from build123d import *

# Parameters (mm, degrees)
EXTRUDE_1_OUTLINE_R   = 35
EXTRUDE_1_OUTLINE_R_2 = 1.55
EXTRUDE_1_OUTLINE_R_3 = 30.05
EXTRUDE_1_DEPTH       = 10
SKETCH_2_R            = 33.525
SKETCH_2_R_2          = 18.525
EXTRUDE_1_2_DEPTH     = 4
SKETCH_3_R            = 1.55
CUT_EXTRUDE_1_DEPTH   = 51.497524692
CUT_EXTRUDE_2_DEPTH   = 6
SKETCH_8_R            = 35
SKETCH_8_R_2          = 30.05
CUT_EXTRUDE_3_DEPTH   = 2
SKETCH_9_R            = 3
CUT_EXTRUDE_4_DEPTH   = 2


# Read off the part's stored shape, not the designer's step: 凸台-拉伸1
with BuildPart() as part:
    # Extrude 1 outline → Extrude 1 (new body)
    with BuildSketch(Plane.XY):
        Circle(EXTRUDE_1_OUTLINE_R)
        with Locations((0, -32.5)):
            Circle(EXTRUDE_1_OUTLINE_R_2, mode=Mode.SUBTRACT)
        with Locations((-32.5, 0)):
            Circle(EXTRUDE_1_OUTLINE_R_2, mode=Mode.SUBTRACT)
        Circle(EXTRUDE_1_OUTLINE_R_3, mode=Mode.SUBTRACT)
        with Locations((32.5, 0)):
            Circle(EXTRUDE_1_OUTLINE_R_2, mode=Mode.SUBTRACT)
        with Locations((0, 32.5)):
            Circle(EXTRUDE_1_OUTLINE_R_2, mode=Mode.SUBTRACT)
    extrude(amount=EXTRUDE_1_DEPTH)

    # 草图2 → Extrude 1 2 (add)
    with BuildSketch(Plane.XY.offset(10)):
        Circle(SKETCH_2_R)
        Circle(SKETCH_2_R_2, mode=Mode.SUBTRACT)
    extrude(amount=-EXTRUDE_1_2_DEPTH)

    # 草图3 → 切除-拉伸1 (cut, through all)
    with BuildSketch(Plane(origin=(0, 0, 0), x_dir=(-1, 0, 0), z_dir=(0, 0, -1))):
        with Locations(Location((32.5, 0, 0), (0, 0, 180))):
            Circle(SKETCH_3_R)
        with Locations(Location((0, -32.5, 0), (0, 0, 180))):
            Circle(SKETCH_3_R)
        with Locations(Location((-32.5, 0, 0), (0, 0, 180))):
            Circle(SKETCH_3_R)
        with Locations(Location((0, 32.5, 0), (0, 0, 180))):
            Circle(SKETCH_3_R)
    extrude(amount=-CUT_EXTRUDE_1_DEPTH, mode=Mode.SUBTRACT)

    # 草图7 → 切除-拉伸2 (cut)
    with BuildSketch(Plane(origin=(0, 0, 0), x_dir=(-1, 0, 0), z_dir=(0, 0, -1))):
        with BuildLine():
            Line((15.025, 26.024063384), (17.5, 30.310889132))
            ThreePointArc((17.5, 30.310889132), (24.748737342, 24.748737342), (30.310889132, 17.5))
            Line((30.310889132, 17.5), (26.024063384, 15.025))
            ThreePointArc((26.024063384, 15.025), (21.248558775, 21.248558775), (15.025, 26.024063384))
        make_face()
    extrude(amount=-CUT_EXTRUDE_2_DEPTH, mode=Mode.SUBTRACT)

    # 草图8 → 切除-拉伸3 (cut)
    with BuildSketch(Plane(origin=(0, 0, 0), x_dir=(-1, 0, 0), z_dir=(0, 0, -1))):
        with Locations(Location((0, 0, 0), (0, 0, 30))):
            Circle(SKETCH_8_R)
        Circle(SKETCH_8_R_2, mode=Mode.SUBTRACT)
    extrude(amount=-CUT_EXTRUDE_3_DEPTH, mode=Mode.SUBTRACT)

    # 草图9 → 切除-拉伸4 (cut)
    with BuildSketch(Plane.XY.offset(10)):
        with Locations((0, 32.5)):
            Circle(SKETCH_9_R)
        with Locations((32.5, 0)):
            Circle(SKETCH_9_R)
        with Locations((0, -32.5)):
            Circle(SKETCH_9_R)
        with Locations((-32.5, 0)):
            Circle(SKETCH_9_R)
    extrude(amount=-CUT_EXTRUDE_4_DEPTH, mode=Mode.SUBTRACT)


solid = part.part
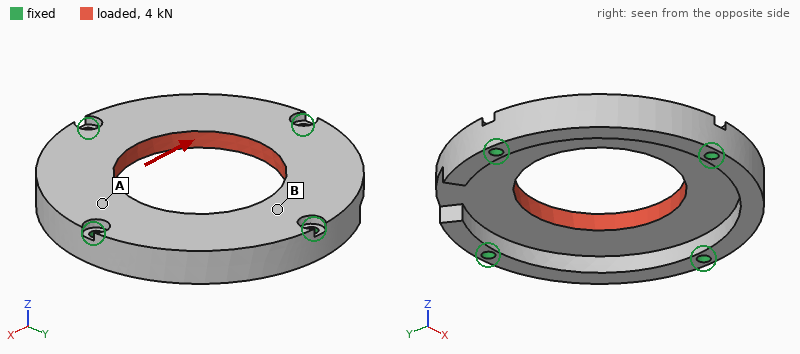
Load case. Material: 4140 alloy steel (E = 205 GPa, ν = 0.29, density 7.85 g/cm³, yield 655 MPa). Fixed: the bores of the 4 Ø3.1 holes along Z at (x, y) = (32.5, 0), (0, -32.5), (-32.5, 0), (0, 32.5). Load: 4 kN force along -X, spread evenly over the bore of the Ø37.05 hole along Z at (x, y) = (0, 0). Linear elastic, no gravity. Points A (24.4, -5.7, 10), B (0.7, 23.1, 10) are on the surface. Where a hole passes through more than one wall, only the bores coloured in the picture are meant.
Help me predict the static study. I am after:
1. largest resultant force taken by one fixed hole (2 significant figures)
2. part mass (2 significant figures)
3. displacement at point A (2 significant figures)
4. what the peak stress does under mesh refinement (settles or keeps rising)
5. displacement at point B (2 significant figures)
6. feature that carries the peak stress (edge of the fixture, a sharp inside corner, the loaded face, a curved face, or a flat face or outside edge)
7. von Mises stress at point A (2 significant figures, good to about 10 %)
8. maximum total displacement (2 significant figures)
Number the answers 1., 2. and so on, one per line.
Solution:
1. 1.1 kN
2. 110 g
3. 2.2 µm
4. keeps rising
5. 1.8 µm
6. edge of the fixture
7. 17 MPa
8. 3.3 µm
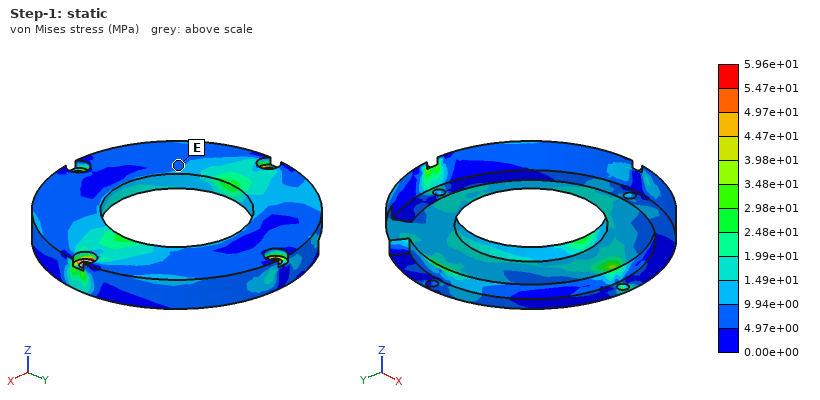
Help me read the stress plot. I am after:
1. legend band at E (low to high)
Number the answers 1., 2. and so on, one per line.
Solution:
1. 4.97e+00 to 9.94e+00 MPa
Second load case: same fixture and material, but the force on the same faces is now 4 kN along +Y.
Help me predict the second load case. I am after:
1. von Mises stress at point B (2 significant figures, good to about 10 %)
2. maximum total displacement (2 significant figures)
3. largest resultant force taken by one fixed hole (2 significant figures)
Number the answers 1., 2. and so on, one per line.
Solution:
1. 21 MPa
2. 3.3 µm
3. 1.1 kN
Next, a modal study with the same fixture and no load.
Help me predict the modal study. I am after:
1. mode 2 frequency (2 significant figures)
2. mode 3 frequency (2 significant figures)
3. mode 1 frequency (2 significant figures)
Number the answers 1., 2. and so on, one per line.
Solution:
1. 11 kHz
2. 12 kHz
3. 11 kHz
